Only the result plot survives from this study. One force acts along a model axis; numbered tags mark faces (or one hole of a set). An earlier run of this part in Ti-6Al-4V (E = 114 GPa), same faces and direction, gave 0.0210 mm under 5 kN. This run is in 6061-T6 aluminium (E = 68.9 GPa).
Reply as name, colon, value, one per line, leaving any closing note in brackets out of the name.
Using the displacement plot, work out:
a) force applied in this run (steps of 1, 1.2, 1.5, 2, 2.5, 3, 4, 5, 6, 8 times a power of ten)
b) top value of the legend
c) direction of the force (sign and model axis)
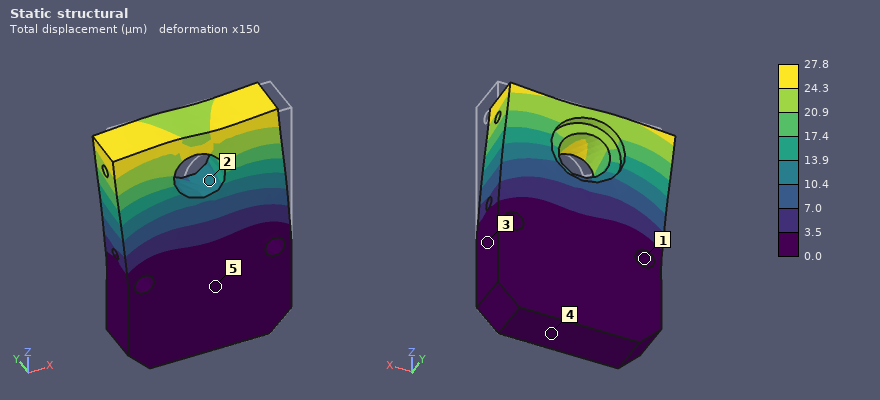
force applied in this run: 4 kN
top value of the legend: 27.8 µm
direction of the force: -X
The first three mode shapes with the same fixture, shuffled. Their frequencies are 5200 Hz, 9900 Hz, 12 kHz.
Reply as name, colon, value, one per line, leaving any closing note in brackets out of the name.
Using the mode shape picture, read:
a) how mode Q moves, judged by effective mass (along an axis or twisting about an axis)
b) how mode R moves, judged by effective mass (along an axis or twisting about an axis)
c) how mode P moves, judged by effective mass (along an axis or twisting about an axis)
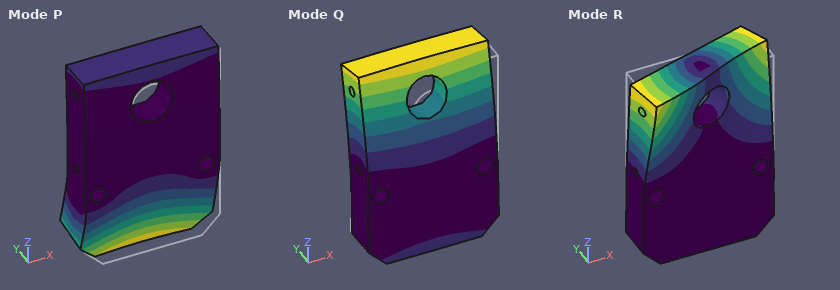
how mode Q moves, judged by effective mass: along Y
how mode R moves, judged by effective mass: twisting about Z
how mode P moves, judged by effective mass: along Y
